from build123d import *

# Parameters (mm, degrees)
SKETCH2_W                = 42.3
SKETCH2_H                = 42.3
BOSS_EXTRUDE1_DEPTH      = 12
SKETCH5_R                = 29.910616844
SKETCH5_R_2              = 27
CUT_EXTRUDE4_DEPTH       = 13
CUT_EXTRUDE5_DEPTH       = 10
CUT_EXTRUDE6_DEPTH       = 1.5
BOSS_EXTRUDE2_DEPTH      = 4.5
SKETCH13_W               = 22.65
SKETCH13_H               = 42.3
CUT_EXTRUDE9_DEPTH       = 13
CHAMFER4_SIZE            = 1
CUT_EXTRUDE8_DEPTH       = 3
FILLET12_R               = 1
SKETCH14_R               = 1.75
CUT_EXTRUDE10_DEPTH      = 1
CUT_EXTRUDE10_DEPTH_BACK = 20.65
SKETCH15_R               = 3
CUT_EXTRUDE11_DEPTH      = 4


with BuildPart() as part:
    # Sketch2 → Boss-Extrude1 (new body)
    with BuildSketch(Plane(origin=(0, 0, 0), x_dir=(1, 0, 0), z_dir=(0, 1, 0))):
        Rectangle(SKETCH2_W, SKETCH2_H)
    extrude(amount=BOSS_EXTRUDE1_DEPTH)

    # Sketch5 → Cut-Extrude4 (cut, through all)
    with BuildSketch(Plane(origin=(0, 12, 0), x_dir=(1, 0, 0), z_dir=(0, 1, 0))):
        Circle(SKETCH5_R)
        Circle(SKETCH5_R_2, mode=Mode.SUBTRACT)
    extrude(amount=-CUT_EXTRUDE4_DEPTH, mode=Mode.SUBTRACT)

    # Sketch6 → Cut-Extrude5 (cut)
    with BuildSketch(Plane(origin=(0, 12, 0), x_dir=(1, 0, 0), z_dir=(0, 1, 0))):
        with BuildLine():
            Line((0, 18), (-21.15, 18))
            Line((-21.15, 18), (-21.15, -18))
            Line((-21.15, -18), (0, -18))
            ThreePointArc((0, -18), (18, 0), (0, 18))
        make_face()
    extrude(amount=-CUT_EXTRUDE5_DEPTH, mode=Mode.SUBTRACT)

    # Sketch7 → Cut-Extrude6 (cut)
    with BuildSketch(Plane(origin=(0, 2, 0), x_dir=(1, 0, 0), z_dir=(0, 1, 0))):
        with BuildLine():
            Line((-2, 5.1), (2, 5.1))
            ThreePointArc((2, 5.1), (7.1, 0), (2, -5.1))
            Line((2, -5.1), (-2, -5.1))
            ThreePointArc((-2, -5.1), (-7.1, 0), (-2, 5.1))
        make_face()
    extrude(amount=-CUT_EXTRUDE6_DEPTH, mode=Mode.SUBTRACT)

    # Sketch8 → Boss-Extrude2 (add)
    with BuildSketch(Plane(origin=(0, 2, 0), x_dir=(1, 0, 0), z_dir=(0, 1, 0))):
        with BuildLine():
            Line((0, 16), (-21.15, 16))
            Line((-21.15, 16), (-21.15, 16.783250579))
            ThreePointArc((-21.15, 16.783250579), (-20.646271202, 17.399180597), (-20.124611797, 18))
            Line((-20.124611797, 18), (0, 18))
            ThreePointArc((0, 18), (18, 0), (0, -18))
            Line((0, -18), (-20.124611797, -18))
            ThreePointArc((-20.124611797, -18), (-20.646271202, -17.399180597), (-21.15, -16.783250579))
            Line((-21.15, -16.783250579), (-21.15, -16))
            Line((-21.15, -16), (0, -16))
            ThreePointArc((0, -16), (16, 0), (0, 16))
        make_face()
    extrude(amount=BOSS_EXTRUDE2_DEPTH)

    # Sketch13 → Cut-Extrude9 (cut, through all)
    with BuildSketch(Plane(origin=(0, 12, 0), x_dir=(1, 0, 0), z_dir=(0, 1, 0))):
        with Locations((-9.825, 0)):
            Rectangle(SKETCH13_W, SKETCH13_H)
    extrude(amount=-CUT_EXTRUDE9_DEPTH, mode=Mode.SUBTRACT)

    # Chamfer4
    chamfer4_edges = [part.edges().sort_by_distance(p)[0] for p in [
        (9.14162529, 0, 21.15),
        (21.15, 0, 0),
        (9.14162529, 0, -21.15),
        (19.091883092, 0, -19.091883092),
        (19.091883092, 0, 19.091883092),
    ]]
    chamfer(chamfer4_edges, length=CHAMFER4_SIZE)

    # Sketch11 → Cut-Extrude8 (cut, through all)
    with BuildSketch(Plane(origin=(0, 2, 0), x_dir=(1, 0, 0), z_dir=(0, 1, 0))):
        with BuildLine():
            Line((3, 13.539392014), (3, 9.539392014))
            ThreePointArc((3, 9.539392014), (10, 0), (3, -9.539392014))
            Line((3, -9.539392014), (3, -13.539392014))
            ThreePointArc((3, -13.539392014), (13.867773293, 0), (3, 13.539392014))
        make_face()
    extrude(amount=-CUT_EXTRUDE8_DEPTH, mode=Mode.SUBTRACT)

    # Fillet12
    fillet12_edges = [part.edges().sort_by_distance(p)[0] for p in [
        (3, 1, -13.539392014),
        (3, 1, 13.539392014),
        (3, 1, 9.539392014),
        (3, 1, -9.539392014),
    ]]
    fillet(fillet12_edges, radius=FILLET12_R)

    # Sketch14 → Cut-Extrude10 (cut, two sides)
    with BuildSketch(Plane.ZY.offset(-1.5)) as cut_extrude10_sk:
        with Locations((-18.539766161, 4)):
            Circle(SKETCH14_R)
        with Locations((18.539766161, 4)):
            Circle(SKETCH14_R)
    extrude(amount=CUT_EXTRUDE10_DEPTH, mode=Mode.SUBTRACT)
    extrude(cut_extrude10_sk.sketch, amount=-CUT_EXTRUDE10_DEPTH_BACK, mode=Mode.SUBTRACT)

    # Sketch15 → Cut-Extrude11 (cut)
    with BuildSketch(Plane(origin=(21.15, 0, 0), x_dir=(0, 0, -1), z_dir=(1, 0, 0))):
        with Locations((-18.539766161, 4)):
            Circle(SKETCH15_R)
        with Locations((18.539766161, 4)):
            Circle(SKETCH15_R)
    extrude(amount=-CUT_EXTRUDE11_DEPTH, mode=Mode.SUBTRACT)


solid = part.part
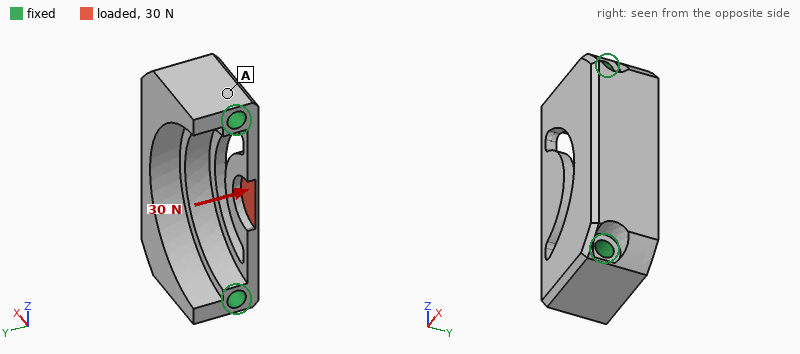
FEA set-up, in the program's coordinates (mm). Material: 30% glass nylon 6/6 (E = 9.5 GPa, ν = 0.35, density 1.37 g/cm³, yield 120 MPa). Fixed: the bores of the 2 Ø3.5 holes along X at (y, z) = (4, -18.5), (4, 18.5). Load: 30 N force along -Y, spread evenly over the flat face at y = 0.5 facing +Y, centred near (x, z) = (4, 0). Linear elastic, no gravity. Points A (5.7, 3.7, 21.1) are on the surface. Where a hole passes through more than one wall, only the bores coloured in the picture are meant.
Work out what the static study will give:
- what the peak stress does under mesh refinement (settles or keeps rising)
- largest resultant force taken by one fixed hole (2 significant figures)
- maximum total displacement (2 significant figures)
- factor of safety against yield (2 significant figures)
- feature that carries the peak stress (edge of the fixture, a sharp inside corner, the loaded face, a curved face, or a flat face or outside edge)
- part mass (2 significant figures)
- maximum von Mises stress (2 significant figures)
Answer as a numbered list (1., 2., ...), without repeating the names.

1. settles
2. 30 N
3. 0.44 mm
4. 1.7
5. a curved face
6. 6.7 g
7. 73 MPa
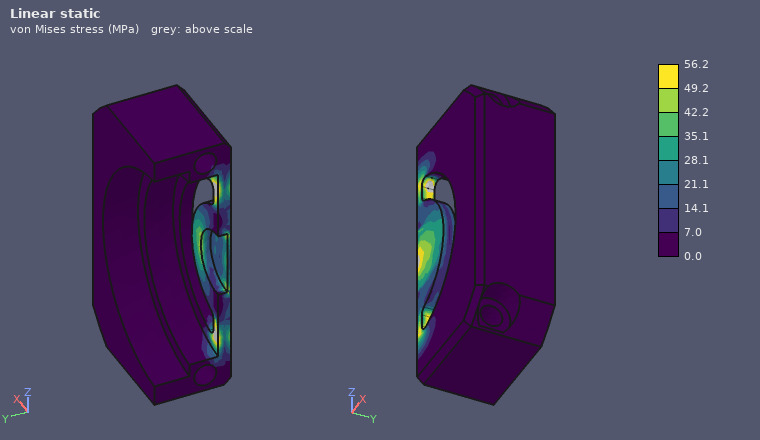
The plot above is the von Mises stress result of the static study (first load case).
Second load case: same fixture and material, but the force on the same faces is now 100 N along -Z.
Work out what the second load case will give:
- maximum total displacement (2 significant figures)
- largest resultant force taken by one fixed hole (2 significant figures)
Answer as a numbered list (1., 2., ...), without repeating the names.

1. 38 µm
2. 50 N
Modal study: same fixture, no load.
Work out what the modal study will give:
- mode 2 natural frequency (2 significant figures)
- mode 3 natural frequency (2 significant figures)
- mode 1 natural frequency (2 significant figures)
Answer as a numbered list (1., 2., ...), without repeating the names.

1. 7800 Hz
2. 8700 Hz
3. 2700 Hz
